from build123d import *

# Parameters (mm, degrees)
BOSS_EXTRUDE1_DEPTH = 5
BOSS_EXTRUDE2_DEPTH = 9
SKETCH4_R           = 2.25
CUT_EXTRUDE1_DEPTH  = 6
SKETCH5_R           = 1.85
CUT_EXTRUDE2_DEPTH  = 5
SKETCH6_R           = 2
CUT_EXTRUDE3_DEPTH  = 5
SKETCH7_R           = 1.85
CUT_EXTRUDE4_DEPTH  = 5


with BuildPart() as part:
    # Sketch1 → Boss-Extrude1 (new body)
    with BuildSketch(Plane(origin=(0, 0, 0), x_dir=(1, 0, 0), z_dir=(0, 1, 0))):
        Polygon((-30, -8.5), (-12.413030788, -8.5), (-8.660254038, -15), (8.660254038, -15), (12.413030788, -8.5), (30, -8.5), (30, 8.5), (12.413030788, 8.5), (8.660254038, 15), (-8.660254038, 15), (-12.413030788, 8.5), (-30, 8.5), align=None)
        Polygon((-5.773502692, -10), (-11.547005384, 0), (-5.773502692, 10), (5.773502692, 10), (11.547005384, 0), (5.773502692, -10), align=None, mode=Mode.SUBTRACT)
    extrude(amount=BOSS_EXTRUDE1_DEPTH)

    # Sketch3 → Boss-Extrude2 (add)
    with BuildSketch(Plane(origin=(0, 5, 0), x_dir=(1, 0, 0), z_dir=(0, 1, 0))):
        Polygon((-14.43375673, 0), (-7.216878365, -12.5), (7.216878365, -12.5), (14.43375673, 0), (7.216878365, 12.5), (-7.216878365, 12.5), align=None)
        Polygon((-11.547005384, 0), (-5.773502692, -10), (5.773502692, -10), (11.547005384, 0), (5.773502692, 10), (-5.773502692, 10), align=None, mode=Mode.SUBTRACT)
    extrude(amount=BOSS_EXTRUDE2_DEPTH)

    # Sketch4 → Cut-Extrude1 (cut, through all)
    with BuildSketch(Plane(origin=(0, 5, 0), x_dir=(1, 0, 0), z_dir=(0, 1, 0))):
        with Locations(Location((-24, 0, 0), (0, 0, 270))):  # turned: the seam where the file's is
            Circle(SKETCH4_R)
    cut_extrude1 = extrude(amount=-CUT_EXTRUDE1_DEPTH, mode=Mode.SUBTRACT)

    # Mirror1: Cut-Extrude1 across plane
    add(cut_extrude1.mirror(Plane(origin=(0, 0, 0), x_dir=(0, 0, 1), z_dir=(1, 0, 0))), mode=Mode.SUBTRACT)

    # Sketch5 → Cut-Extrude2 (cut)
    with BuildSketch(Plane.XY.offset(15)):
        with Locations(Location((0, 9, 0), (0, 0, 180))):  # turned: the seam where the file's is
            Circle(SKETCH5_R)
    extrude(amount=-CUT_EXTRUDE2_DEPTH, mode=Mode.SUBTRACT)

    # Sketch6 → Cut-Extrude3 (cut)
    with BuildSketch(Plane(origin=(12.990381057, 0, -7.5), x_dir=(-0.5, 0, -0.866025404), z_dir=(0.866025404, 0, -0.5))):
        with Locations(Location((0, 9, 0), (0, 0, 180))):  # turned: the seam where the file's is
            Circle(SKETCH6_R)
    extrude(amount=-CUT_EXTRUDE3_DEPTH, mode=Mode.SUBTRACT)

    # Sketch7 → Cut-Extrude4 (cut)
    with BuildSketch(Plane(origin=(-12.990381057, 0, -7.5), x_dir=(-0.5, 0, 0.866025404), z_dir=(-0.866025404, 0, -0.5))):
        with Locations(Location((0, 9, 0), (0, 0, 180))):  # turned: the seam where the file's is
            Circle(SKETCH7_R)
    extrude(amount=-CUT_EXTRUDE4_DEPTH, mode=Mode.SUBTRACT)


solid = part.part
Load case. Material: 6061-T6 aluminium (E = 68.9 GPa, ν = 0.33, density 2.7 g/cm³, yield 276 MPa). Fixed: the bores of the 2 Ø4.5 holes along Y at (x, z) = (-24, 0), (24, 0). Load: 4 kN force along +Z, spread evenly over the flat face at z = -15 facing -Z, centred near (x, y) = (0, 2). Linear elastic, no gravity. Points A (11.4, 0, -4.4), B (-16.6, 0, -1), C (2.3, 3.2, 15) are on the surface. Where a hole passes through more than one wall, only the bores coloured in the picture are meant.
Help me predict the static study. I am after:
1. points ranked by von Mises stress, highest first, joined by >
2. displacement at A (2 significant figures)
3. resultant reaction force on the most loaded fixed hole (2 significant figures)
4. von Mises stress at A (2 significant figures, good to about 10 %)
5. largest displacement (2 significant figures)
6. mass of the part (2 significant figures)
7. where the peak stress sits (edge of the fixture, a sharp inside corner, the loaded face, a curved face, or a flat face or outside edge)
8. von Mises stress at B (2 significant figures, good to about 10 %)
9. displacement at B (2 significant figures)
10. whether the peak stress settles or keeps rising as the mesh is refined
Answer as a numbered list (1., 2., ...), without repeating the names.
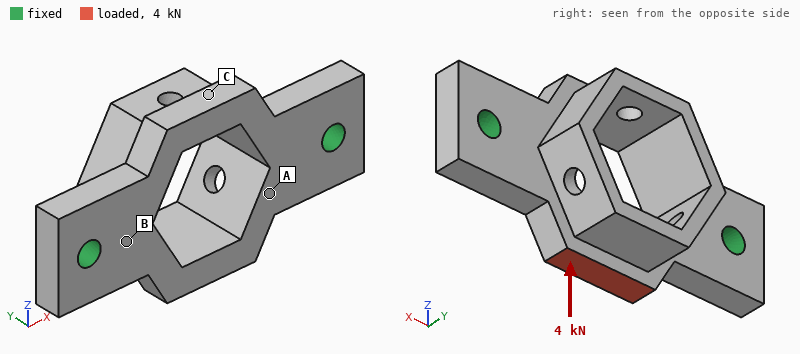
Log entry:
1. A > B > C
2. 26 µm
3. 2.5 kN
4. 93 MPa
5. 67 µm
6. 17 g
7. a sharp inside corner
8. 59 MPa
9. 13 µm
10. keeps rising
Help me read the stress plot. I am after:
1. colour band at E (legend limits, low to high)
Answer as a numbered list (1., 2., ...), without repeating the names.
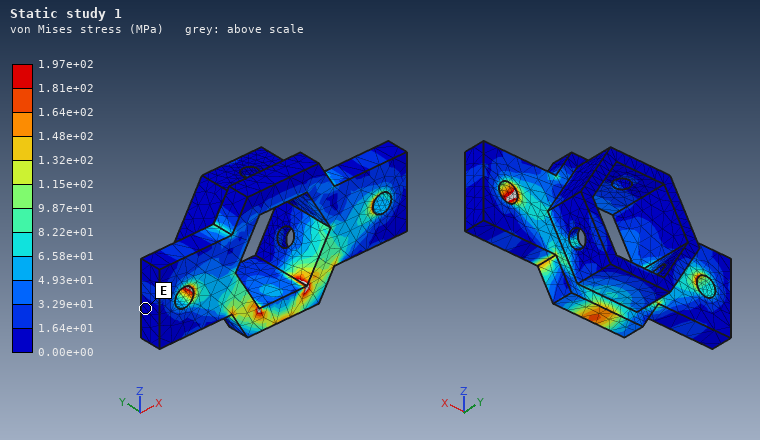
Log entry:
1. 0.00e+00 to 1.64e+01 MPa
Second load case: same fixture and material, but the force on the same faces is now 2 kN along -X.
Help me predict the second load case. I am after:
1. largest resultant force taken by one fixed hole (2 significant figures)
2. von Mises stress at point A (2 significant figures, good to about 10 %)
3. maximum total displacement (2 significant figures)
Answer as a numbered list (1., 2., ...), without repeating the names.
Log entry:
1. 1.2 kN
2. 16 MPa
3. 24 µm
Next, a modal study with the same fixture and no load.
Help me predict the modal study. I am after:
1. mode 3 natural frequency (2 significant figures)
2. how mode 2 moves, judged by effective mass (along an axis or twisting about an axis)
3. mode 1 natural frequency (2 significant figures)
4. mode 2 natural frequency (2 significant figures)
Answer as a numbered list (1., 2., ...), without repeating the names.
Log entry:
1. 17 kHz
2. along Y
3. 7300 Hz
4. 9100 Hz
